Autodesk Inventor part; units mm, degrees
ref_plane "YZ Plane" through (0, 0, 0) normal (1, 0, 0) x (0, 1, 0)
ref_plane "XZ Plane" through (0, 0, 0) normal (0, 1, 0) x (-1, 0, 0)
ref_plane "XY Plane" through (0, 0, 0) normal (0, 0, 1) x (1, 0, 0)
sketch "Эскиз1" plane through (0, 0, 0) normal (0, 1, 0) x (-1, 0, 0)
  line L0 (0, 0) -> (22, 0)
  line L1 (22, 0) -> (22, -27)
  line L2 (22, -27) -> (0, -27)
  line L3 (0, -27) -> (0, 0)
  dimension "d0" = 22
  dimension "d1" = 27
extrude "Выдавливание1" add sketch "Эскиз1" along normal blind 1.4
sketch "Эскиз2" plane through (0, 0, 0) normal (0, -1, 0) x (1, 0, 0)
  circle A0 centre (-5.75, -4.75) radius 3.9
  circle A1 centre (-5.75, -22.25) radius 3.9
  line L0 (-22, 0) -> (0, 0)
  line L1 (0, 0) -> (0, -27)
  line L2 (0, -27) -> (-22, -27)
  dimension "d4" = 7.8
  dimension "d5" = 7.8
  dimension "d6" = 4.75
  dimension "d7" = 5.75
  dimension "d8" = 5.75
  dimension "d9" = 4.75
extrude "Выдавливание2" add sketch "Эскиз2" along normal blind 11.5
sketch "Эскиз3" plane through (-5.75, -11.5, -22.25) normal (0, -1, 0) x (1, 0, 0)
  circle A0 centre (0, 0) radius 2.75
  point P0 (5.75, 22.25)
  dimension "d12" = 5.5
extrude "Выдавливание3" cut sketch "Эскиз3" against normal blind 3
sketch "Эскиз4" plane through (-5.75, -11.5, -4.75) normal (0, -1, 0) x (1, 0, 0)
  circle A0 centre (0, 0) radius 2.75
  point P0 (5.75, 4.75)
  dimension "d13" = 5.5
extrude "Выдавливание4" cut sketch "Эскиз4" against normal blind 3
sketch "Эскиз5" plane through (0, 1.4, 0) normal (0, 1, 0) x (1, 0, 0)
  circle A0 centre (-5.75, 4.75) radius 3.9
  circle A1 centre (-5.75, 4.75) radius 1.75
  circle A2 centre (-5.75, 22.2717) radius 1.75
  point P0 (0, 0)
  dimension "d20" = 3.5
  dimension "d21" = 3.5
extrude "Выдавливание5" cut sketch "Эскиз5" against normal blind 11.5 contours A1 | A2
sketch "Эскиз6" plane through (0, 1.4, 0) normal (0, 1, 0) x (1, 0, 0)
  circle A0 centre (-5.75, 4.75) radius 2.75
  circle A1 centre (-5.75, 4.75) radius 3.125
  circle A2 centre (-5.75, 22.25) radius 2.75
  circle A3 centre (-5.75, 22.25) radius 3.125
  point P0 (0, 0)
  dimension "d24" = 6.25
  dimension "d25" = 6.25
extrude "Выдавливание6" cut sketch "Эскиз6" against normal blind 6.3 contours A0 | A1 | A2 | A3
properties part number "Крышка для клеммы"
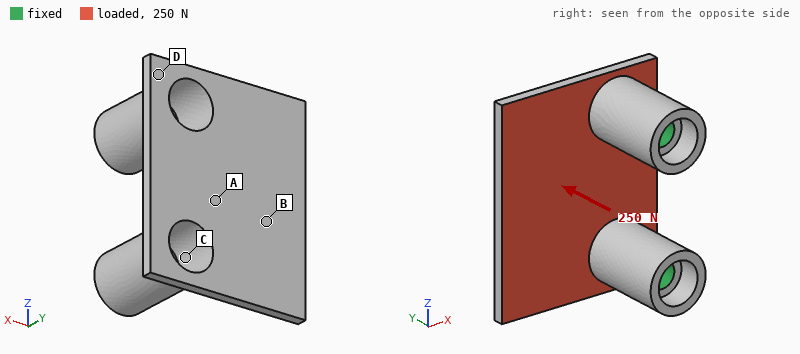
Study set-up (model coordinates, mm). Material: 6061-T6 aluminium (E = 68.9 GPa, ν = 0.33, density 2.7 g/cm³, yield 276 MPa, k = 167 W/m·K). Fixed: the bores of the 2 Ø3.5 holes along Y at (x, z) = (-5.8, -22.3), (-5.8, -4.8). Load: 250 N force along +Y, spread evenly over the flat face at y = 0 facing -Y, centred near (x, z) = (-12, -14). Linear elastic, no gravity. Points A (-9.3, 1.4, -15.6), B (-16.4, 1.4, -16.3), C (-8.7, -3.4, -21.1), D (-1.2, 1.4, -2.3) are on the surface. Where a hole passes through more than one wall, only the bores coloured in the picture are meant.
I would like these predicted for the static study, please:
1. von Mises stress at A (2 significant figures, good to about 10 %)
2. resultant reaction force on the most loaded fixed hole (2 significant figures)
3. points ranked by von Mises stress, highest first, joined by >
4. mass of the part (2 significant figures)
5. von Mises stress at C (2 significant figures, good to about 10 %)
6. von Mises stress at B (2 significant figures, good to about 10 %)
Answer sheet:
90 MPa
130 N
A > C > B > D
3.6 g
55 MPa
29 MPa
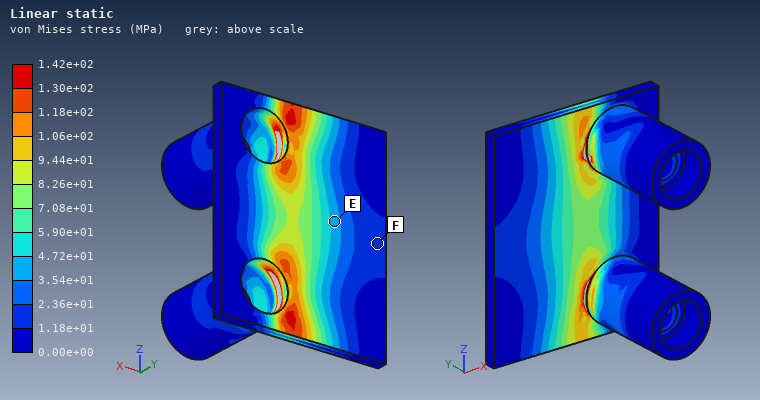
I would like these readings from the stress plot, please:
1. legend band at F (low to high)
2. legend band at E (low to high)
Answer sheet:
1.18e+01 to 2.36e+01 MPa
3.54e+01 to 4.72e+01 MPa
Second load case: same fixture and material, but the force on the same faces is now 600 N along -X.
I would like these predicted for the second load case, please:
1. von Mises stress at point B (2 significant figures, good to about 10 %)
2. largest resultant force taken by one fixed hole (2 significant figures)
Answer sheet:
11 MPa
300 N
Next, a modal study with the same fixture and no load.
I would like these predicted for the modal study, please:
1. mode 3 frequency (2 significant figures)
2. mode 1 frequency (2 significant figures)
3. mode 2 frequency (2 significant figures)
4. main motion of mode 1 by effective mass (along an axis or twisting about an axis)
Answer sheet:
16 kHz
4900 Hz
8400 Hz
along Y
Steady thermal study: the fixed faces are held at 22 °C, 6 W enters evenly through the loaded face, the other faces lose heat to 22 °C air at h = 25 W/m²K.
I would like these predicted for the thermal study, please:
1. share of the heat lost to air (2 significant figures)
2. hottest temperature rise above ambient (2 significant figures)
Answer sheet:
3.6 %
13 K
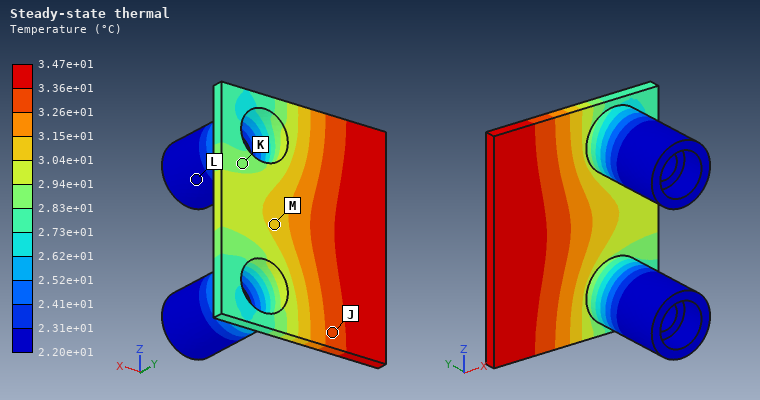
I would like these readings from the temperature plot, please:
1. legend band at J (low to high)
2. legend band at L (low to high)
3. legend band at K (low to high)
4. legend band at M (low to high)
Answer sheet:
3.26e+01 to 3.36e+01 °C
2.20e+01 to 2.31e+01 °C
2.83e+01 to 2.94e+01 °C
3.04e+01 to 3.15e+01 °C
